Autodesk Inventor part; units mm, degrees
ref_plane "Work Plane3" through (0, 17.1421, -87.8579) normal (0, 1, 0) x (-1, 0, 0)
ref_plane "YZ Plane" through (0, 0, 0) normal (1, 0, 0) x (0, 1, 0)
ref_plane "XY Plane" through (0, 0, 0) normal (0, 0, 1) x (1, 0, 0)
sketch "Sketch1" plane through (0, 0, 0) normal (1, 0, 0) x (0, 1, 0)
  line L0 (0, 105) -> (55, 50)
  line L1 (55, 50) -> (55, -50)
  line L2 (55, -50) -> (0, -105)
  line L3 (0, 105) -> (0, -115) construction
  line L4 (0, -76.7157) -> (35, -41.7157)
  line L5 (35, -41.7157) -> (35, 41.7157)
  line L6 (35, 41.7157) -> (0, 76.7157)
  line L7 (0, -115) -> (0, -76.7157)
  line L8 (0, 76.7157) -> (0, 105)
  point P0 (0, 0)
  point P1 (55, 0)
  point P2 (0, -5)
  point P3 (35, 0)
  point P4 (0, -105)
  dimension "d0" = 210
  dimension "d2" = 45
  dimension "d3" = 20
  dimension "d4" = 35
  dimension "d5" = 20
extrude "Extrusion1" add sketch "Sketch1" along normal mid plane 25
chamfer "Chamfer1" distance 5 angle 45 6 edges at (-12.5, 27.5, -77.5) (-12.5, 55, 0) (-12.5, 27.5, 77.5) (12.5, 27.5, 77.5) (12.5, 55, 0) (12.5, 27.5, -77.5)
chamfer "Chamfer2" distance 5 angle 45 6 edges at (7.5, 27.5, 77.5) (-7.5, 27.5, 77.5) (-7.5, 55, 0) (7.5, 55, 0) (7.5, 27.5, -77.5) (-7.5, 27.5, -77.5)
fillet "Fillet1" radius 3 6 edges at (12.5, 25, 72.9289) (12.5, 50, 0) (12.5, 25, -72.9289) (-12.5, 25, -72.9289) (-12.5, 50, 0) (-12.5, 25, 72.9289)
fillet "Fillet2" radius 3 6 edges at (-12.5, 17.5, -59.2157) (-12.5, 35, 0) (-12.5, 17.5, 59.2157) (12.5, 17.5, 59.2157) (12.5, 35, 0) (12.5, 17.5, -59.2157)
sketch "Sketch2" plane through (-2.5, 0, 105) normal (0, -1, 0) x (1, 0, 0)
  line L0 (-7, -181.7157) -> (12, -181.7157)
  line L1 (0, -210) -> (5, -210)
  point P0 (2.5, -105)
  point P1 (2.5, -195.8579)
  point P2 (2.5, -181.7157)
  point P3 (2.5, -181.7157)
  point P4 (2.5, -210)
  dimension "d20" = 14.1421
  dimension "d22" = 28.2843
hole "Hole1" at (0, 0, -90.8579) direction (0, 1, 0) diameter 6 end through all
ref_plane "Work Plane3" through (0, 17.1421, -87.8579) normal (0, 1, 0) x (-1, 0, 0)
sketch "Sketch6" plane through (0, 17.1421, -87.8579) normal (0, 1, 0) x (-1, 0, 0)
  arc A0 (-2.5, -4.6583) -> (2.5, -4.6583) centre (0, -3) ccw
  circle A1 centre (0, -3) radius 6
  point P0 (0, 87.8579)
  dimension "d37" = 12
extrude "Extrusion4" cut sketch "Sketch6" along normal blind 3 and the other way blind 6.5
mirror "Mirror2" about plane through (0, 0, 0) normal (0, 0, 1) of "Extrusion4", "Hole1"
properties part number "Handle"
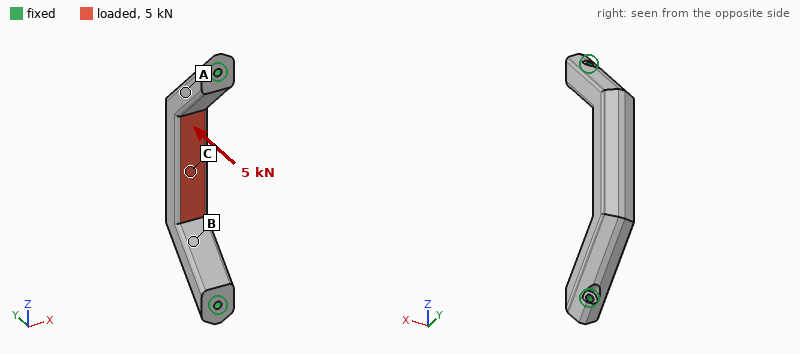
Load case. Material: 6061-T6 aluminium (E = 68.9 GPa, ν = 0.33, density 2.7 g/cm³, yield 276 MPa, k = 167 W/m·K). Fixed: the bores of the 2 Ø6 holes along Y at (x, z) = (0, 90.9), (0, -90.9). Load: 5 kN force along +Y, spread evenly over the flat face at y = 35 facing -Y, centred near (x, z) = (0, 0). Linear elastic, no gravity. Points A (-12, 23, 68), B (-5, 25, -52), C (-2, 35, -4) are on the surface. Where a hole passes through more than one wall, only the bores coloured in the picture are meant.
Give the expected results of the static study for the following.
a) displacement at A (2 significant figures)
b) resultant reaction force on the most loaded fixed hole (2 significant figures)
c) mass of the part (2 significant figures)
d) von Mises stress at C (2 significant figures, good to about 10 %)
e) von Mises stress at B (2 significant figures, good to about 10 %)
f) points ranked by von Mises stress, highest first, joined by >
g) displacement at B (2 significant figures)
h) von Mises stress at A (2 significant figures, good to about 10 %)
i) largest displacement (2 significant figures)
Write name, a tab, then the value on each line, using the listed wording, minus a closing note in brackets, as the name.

displacement at A	8.1 µm
resultant reaction force on the most loaded fixed hole	4.2 kN
mass of the part	260 g
von Mises stress at C	16 MPa
von Mises stress at B	21 MPa
points ranked by von Mises stress, highest first, joined by >	B > C > A
displacement at B	15 µm
von Mises stress at A	10 MPa
largest displacement	54 µm
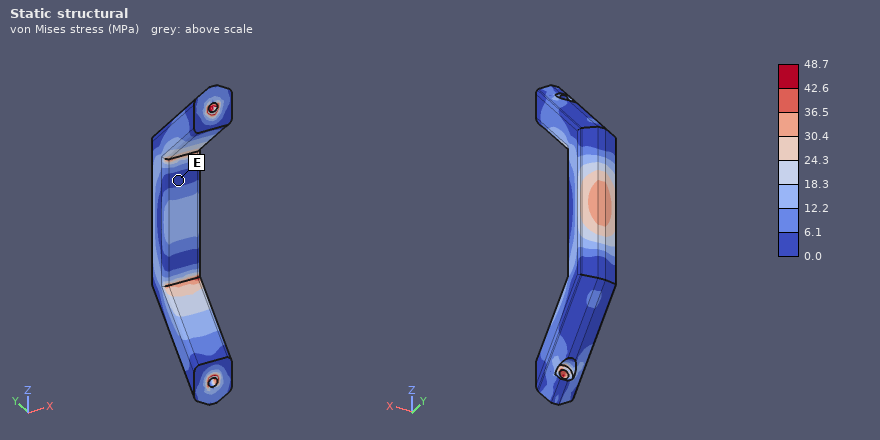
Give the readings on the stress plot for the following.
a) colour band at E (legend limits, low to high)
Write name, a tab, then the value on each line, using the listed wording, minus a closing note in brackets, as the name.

colour band at E	0.0 to 6.1 MPa
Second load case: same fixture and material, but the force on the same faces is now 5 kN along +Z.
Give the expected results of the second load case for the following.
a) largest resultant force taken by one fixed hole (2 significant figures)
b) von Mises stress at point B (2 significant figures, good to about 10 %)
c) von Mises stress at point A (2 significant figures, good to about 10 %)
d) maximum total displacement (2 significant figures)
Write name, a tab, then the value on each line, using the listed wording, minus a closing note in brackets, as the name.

largest resultant force taken by one fixed hole	2.6 kN
von Mises stress at point B	24 MPa
von Mises stress at point A	10 MPa
maximum total displacement	57 µm
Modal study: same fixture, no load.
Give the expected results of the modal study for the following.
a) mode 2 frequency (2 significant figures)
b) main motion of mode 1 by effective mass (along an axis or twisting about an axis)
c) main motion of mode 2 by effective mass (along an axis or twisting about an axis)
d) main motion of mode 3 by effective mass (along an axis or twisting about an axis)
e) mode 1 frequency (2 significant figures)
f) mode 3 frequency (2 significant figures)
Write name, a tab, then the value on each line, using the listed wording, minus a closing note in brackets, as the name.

mode 2 frequency	3600 Hz
main motion of mode 1 by effective mass	along X
main motion of mode 2 by effective mass	along Z
main motion of mode 3 by effective mass	twisting about Y
mode 1 frequency	1500 Hz
mode 3 frequency	4300 Hz
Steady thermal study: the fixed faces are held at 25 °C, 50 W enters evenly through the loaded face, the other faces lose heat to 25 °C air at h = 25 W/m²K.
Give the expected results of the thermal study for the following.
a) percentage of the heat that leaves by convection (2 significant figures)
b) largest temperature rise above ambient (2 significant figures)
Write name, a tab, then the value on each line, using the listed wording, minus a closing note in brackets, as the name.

percentage of the heat that leaves by convection	12 %
largest temperature rise above ambient	28 K
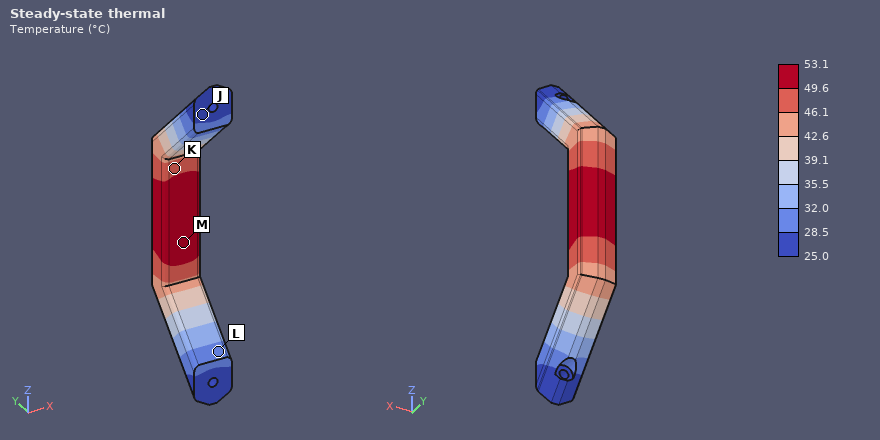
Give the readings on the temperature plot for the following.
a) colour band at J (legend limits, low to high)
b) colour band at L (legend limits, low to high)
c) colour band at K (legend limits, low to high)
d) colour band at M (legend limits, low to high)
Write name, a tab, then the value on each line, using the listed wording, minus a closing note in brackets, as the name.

colour band at J	25.0 to 28.5 °C
colour band at L	28.5 to 32.0 °C
colour band at K	46.1 to 49.6 °C
colour band at M	49.6 to 53.1 °C
